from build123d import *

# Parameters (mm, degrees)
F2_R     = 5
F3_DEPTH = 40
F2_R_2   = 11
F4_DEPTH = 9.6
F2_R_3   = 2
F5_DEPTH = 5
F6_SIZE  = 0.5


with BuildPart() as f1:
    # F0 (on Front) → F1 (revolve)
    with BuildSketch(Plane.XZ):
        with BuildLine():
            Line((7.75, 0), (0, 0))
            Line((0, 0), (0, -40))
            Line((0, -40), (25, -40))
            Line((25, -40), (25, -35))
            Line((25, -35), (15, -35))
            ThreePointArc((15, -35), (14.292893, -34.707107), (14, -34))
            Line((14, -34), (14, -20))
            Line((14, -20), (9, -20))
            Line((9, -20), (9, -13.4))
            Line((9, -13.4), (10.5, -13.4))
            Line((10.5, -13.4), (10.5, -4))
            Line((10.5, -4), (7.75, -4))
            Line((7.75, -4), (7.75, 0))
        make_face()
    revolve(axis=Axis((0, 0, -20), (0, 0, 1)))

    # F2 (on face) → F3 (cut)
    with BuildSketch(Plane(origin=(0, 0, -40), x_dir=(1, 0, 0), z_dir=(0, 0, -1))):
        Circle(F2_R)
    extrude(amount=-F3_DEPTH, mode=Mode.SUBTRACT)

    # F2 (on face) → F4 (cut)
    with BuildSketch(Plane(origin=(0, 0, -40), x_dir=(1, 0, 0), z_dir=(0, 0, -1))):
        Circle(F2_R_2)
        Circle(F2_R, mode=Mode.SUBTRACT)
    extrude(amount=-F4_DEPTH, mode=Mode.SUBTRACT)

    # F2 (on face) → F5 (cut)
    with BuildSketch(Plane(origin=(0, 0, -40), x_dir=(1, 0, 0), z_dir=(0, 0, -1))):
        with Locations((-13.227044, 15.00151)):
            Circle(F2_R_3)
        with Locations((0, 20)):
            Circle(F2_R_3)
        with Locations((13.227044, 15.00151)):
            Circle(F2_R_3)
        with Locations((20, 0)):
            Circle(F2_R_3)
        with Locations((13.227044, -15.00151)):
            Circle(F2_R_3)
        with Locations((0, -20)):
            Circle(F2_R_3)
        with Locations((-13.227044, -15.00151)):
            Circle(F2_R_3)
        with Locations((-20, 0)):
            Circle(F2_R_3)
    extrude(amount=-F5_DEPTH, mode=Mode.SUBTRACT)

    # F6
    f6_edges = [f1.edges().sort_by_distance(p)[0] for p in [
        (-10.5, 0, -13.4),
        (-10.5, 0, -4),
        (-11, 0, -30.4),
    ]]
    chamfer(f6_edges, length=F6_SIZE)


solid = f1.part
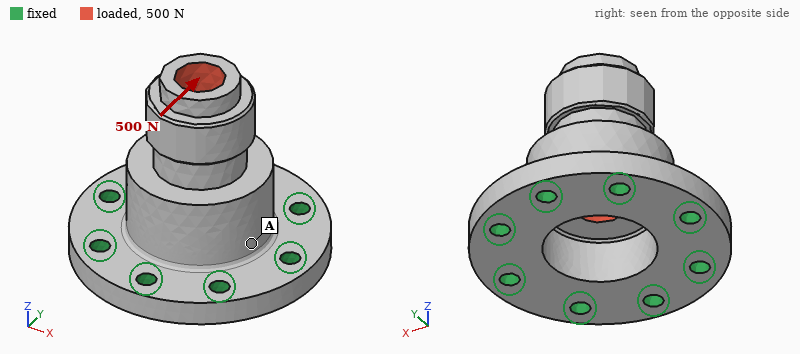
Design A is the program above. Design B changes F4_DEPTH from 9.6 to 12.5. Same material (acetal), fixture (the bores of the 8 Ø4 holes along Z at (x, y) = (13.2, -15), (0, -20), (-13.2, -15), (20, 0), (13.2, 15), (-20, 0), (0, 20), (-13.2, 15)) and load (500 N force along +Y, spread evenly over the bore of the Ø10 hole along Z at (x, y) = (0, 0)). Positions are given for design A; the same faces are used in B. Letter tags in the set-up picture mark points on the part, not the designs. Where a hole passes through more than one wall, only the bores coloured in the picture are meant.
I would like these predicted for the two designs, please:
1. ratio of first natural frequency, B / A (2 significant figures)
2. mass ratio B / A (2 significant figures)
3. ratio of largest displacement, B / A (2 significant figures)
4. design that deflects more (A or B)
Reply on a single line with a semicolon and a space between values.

0.95; 0.95; 1.2; B
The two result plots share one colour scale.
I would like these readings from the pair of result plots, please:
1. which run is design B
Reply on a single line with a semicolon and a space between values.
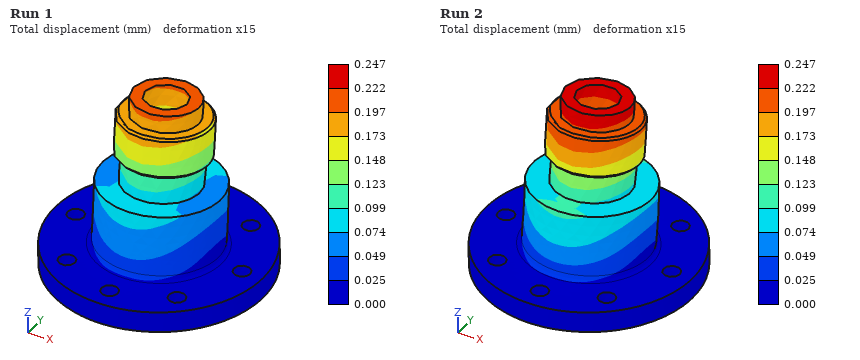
Run 2
